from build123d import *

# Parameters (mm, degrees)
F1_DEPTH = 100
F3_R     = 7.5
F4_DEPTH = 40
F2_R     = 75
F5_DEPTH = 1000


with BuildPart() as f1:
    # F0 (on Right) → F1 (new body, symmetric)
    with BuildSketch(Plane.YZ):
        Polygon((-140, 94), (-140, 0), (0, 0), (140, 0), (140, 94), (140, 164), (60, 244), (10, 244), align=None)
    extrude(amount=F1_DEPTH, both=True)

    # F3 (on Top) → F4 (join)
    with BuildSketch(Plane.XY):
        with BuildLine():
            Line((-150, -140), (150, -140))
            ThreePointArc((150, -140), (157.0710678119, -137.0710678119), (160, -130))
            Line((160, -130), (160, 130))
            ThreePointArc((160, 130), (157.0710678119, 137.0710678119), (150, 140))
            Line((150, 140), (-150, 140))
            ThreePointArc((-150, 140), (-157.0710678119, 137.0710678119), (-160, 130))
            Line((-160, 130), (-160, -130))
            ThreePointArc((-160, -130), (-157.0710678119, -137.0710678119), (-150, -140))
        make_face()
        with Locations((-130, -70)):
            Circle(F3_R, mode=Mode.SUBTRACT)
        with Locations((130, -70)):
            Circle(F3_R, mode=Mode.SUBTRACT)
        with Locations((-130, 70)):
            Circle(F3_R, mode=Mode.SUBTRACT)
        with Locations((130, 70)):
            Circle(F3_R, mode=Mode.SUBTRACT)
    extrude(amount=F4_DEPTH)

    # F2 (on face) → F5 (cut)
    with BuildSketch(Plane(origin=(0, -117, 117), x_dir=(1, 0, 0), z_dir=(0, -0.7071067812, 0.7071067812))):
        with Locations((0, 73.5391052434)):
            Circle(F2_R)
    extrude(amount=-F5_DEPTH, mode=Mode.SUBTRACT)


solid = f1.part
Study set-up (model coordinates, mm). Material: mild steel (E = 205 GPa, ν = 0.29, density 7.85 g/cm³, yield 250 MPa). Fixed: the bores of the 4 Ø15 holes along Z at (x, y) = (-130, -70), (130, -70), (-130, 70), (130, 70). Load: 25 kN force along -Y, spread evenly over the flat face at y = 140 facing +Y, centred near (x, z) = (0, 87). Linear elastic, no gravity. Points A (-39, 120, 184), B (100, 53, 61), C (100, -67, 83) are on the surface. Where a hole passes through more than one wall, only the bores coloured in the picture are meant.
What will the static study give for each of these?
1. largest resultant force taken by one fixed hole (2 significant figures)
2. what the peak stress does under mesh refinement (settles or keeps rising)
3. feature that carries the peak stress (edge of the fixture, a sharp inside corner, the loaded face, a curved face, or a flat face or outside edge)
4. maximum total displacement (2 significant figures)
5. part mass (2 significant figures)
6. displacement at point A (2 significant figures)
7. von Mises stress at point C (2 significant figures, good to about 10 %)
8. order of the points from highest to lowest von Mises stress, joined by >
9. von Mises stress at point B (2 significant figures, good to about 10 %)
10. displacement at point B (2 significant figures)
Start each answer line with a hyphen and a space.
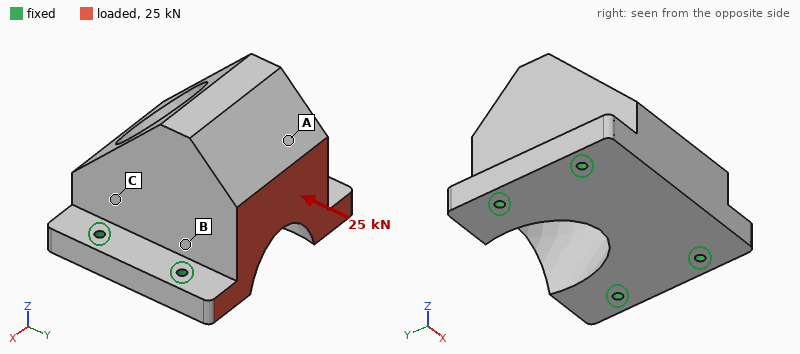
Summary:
- 8.9 kN
- keeps rising
- edge of the fixture
- 9.7 µm
- 63 kg
- 8.6 µm
- 2.1 MPa
- B > C > A
- 4.1 MPa
- 3.2 µm
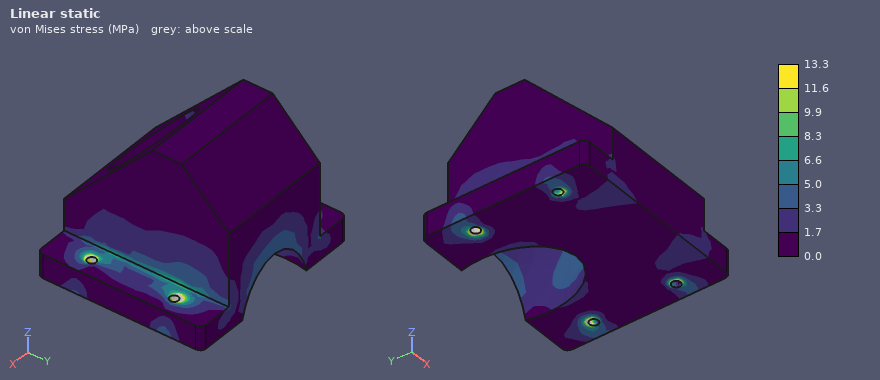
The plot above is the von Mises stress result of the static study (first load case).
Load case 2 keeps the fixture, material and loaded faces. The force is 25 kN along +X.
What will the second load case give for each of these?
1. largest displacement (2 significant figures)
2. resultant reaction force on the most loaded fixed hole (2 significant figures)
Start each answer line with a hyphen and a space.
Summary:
- 9.5 µm
- 14 kN
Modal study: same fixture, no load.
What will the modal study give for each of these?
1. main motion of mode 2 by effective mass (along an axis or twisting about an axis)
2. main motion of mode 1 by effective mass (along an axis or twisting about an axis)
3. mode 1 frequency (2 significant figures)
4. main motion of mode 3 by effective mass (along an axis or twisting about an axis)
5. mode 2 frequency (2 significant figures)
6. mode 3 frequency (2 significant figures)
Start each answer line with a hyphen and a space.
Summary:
- along X
- along Y
- 1100 Hz
- along Z
- 1400 Hz
- 2100 Hz
